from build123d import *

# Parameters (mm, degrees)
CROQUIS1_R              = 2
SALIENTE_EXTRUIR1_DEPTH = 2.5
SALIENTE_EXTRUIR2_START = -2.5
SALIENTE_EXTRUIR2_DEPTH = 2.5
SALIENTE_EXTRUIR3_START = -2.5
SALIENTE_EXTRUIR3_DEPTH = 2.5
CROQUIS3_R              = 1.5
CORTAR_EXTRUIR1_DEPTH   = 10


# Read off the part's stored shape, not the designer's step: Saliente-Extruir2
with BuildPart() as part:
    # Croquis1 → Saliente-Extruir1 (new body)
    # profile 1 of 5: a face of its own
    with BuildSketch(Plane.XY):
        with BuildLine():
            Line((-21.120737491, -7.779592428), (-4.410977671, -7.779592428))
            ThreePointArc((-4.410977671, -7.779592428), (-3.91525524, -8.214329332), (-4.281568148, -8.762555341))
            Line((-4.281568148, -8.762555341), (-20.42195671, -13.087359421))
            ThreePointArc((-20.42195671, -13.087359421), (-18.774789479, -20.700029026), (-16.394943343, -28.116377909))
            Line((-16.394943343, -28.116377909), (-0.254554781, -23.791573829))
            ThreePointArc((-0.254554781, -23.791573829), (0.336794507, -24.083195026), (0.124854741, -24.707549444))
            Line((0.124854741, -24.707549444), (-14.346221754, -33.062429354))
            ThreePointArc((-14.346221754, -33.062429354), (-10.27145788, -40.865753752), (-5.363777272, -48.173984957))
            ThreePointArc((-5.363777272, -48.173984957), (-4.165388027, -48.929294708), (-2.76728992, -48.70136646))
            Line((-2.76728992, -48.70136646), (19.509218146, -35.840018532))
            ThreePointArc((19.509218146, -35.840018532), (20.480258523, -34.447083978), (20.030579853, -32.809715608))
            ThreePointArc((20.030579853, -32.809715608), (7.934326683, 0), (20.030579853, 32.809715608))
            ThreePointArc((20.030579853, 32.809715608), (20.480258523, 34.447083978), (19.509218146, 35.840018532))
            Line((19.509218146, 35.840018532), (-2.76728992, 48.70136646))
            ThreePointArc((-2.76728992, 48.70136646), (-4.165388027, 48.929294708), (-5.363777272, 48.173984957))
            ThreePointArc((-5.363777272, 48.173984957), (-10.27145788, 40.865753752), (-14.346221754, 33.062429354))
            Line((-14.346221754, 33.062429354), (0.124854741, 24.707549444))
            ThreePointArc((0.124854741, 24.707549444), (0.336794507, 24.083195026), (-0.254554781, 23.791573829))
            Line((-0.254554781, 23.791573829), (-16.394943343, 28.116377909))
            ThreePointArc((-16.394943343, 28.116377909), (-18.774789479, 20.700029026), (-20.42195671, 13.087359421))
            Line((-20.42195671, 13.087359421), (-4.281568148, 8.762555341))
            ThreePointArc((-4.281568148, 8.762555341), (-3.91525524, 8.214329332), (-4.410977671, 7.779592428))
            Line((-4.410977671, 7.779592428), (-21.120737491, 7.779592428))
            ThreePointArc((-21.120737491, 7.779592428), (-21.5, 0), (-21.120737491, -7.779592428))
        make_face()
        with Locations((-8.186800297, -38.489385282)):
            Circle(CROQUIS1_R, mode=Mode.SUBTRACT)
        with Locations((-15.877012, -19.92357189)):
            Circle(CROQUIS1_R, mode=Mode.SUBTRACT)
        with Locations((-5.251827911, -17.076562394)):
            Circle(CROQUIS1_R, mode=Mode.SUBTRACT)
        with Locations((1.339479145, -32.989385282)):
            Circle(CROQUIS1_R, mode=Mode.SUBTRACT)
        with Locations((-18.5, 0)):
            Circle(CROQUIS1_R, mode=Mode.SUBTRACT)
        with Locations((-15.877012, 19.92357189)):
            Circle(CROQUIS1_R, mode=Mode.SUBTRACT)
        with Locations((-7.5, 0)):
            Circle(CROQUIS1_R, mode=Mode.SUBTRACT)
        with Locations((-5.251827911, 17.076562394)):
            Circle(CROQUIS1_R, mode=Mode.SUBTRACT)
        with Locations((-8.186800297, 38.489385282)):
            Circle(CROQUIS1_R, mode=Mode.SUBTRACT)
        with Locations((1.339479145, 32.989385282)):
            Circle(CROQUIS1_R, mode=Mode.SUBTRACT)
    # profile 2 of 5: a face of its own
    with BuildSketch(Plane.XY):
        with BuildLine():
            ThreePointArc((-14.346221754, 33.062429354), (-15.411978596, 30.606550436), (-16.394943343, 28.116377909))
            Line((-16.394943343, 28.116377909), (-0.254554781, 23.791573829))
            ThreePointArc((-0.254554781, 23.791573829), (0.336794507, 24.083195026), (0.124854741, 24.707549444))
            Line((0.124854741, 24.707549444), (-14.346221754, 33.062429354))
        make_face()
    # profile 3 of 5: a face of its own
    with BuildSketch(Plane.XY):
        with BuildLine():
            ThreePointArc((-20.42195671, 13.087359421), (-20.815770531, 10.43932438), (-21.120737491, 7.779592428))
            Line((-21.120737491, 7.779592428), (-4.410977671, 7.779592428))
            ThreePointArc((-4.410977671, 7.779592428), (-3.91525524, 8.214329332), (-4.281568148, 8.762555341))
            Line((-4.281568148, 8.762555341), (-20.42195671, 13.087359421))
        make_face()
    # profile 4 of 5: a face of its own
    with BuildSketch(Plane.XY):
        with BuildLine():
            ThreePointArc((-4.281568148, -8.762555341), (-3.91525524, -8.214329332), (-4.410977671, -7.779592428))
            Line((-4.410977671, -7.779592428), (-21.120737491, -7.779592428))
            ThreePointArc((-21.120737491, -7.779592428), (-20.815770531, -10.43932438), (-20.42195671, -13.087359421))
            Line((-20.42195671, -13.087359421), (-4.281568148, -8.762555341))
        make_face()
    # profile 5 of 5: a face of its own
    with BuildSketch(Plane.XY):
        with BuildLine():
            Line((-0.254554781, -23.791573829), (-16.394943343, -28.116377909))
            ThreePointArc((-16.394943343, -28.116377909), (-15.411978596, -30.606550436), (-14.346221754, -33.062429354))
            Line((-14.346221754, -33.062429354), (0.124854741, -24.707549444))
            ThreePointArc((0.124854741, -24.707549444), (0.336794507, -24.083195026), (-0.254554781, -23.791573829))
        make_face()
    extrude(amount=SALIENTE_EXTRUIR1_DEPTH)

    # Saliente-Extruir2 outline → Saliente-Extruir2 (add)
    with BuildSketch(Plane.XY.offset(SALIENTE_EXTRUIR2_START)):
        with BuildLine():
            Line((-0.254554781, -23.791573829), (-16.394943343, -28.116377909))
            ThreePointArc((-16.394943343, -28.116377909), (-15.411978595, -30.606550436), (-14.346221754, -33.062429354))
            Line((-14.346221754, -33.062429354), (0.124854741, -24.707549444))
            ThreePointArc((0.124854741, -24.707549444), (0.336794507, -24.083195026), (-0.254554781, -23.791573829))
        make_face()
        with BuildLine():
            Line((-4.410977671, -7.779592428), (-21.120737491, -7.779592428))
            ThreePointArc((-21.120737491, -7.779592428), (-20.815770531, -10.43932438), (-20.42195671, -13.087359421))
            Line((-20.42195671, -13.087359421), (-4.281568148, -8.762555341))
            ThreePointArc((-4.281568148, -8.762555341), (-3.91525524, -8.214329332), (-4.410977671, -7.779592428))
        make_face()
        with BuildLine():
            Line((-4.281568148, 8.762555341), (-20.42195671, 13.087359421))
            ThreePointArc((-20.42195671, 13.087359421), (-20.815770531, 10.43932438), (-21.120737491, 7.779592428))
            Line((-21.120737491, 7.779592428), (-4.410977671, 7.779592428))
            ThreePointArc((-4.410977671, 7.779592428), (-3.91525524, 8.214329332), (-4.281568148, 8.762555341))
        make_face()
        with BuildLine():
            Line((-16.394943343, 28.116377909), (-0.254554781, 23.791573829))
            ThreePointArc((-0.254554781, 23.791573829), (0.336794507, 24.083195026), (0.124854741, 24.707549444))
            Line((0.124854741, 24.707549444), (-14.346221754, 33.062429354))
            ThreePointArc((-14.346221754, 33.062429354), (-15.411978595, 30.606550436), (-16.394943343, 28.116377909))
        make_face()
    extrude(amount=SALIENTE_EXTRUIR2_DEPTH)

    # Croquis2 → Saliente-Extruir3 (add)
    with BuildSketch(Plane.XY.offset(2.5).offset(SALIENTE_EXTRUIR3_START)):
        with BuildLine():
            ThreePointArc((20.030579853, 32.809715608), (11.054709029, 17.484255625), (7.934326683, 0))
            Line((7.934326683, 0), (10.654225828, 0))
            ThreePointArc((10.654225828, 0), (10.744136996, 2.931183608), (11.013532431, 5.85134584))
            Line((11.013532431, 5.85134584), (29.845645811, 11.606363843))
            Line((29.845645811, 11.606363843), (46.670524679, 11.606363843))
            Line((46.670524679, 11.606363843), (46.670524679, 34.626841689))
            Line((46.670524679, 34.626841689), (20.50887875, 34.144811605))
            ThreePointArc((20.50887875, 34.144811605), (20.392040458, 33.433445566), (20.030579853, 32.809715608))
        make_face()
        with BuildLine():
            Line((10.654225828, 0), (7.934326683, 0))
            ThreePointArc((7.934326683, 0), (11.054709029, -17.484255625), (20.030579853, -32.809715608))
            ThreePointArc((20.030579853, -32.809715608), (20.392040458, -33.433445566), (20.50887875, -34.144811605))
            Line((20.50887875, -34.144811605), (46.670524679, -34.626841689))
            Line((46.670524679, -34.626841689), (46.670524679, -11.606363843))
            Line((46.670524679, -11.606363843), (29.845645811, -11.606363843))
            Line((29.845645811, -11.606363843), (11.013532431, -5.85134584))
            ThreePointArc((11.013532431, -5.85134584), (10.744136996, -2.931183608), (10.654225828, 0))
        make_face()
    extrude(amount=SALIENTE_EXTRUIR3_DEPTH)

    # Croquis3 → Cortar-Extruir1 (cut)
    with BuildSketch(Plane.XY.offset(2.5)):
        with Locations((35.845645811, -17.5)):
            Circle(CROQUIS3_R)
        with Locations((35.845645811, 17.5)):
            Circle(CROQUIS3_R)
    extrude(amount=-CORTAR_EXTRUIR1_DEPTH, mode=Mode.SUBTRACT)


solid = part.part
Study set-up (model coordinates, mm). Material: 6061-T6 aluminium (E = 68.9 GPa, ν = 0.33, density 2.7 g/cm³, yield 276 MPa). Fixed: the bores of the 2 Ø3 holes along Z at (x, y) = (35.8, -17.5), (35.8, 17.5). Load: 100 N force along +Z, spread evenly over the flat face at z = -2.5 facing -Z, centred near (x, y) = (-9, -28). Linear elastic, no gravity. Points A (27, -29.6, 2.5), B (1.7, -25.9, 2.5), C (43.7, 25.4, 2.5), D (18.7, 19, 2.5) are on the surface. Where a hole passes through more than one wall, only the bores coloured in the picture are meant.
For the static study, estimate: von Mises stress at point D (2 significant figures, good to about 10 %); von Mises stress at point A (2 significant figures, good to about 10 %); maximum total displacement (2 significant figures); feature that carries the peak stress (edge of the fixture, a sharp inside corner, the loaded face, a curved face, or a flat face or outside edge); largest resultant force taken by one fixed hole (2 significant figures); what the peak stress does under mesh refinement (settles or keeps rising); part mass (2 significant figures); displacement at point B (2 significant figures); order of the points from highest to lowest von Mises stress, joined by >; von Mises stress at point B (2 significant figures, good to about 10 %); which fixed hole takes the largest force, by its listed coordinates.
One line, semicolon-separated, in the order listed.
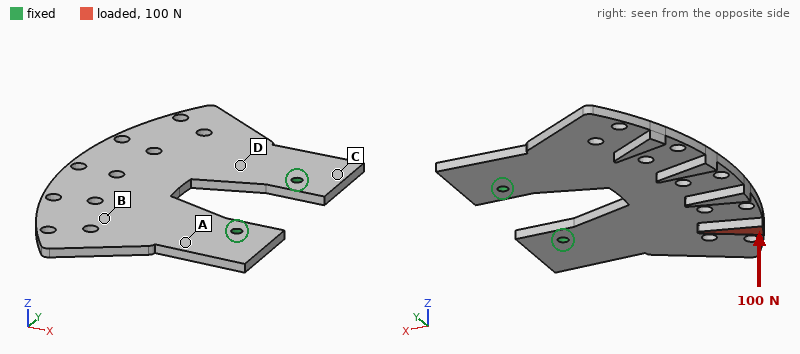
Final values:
45 MPa; 86 MPa; 1.2 mm; edge of the fixture; 91 N; keeps rising; 30 g; 0.70 mm; A > D > B > C; 26 MPa; (35.8, -17.5)
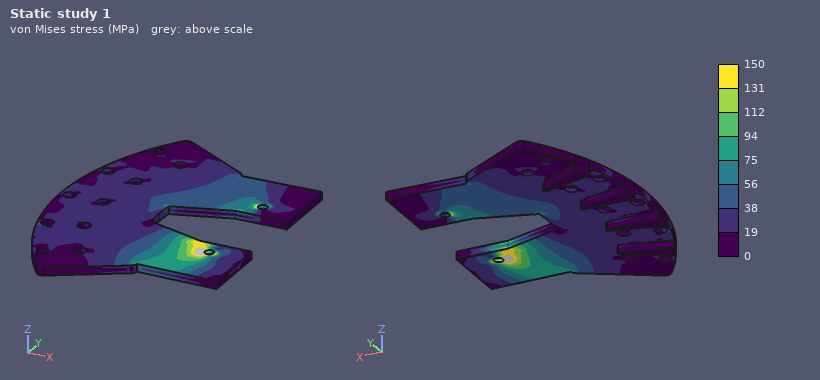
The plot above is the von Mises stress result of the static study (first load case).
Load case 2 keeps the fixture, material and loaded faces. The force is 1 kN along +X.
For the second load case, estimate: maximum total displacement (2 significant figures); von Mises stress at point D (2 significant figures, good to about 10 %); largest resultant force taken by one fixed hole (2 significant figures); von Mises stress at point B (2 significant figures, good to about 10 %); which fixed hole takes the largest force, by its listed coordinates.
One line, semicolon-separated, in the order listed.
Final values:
1.4 mm; 58 MPa; 1.2 kN; 74 MPa; (35.8, -17.5)
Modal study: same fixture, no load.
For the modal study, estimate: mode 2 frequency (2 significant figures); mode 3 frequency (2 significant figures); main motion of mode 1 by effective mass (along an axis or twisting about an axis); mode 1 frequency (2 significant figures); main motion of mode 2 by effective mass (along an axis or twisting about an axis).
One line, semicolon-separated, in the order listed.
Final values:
940 Hz; 2000 Hz; along Z; 490 Hz; twisting about X
